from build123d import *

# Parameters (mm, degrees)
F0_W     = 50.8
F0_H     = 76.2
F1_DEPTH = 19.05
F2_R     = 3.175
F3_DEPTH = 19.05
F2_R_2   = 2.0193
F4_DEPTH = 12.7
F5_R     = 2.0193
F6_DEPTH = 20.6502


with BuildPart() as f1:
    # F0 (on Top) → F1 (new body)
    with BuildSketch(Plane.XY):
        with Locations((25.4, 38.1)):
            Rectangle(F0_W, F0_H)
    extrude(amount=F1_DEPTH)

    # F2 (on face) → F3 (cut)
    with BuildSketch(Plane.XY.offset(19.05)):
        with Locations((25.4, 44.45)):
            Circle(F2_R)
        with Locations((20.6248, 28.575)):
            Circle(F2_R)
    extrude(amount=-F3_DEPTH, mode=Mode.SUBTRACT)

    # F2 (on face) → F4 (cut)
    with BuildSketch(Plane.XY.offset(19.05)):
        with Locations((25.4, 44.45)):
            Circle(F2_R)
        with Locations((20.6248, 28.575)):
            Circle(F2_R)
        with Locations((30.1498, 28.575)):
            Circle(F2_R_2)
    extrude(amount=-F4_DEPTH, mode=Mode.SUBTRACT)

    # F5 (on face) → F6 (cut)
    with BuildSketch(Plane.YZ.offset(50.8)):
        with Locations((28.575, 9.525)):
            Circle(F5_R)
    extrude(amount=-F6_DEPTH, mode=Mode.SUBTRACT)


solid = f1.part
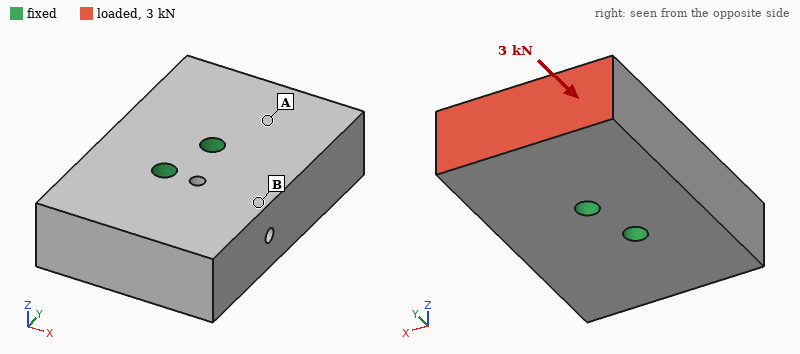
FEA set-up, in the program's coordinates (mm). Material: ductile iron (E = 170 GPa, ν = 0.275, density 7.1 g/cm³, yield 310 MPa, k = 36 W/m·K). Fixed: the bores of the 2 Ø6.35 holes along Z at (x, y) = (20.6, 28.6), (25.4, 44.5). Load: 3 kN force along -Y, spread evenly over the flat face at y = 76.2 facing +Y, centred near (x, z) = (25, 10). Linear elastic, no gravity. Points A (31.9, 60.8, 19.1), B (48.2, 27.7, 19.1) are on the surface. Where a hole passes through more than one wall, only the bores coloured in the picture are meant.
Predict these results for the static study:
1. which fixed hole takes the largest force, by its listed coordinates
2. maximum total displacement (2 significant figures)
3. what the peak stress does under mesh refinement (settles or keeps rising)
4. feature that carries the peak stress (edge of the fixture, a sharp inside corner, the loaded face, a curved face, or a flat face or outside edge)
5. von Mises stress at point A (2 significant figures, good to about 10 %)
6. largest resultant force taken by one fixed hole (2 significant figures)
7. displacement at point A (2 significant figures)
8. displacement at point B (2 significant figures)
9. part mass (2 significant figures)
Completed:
(25.4, 44.5)
1.1 µm
keeps rising
edge of the fixture
3.9 MPa
2.1 kN
0.55 µm
0.41 µm
510 g
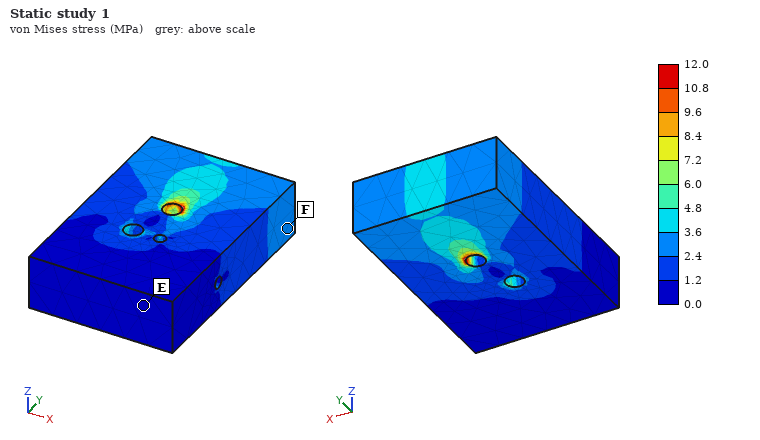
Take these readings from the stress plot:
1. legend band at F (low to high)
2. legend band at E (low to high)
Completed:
2.4 to 3.6 MPa
0.0 to 1.2 MPa
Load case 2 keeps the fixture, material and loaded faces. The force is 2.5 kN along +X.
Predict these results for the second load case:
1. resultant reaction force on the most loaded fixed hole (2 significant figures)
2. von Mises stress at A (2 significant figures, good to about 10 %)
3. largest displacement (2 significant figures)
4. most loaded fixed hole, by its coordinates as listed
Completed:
5.6 kN
5.8 MPa
7.0 µm
(25.4, 44.5)
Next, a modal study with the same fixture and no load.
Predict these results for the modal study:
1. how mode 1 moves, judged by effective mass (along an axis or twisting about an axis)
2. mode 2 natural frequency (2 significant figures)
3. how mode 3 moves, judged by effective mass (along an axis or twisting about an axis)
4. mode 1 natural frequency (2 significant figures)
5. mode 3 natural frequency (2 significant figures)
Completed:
twisting about Z
9100 Hz
along Z
8700 Hz
10 kHz
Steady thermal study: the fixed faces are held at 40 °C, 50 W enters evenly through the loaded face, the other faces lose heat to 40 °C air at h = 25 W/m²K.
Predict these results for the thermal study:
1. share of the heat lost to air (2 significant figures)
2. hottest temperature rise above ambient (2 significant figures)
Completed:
8.2 %
51 K
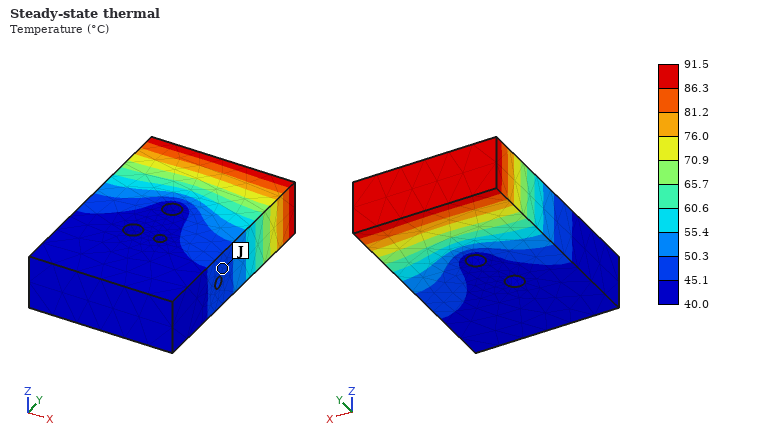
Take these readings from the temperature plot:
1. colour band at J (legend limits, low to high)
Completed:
45.1 to 50.3 °C
